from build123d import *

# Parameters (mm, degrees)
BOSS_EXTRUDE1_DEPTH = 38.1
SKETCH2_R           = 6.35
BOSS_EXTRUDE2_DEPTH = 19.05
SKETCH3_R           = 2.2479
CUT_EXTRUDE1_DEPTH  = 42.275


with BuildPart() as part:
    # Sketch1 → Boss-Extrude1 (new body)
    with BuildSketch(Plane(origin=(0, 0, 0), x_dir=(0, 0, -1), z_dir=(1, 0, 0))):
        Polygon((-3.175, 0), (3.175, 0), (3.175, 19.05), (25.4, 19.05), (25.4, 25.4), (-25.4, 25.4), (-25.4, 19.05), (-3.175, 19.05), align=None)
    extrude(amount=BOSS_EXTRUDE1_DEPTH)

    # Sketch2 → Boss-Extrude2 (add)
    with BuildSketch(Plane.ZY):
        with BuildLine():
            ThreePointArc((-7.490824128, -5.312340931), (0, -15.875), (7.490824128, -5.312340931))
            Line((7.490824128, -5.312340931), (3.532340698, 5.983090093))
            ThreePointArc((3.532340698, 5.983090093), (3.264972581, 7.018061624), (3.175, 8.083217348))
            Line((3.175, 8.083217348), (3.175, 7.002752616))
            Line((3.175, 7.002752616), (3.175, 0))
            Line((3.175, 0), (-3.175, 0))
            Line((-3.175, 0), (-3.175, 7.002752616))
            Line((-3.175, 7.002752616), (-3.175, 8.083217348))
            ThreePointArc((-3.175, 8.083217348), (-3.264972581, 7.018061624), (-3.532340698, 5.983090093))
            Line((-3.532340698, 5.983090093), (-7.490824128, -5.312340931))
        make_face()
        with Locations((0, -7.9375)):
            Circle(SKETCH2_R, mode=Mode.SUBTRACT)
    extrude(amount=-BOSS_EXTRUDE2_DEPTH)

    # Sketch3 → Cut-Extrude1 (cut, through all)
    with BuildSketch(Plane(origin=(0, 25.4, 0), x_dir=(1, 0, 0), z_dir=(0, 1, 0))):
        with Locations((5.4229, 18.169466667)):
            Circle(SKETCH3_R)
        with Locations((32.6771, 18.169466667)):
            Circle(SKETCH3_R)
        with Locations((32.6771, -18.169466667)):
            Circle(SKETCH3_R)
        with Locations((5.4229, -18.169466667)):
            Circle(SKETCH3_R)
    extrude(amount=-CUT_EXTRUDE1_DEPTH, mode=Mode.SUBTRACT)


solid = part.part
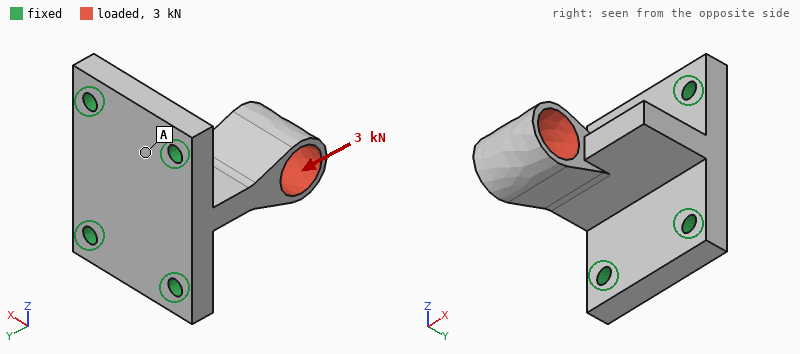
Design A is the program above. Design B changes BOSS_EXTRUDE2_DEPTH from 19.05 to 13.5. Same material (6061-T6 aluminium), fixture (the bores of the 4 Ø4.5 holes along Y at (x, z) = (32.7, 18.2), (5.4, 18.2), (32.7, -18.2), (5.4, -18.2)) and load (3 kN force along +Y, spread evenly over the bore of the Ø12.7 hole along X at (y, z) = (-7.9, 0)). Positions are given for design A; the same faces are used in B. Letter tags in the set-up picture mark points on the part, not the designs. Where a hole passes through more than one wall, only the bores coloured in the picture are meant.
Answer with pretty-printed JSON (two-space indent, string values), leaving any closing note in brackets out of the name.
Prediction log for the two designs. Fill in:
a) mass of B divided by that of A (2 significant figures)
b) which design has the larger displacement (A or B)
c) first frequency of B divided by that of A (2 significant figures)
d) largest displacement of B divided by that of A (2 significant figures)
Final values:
{
  "mass of B divided by that of A": "0.97",
  "which design has the larger displacement": "B",
  "first frequency of B divided by that of A": "1.1",
  "largest displacement of B divided by that of A": "1.3"
}
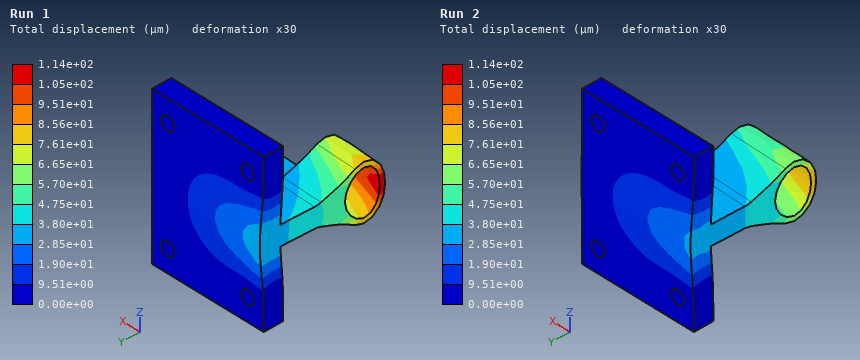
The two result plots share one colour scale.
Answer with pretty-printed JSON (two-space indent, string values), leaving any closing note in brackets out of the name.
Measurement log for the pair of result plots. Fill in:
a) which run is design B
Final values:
{
  "which run is design B": "Run 1"
}
